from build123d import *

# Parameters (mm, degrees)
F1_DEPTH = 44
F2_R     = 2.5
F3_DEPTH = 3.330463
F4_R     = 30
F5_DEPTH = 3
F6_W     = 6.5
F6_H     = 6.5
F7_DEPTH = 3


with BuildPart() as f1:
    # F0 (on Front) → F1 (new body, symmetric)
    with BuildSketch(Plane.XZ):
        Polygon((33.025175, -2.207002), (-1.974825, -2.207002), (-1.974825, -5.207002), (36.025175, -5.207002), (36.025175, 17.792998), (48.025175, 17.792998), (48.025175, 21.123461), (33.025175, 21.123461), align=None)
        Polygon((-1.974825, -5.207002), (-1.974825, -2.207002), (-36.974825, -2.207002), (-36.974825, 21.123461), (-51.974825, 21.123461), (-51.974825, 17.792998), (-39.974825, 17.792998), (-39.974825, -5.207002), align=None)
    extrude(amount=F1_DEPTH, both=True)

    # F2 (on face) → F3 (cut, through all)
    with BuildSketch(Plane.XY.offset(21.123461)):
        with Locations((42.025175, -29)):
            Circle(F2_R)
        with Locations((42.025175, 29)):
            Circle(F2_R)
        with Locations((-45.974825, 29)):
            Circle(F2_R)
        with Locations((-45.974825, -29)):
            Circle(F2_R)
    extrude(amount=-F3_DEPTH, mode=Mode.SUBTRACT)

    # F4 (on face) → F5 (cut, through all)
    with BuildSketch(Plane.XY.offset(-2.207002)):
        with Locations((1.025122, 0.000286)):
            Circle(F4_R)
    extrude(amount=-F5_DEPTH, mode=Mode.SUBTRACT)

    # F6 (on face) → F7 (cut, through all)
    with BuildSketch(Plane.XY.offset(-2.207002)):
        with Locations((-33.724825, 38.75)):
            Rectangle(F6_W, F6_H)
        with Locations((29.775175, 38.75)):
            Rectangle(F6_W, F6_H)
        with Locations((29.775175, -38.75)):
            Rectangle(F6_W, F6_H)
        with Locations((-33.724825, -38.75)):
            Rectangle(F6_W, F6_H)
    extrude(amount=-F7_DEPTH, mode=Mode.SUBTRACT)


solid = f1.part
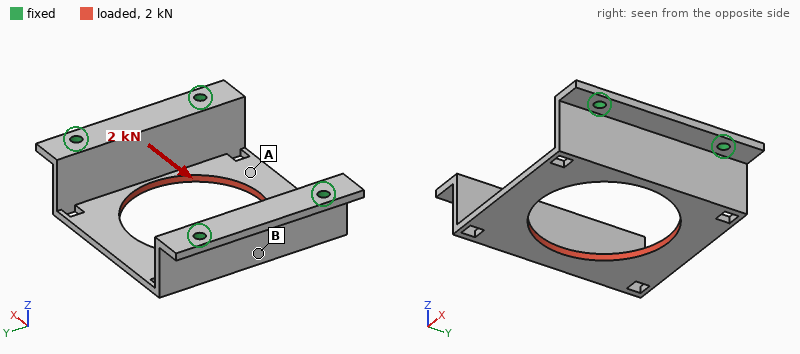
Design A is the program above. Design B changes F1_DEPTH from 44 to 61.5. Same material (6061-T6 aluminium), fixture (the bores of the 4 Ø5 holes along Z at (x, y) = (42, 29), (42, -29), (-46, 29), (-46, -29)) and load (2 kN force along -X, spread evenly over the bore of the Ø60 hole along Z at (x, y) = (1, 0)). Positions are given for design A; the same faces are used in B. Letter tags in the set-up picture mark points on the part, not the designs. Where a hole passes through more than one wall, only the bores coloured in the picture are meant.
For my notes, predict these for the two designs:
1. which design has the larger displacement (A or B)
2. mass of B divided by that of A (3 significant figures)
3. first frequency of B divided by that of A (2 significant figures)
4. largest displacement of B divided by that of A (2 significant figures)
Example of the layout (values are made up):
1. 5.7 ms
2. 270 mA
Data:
1. A
2. 1.52
3. 0.92
4. 0.73
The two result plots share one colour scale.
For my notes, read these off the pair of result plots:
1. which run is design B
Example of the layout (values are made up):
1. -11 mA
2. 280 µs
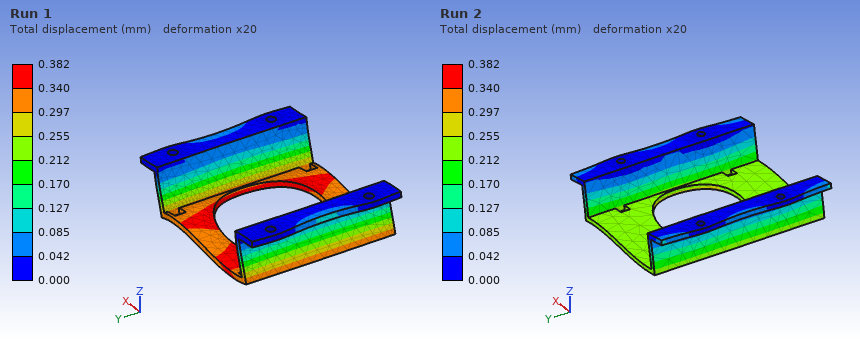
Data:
1. Run 2
